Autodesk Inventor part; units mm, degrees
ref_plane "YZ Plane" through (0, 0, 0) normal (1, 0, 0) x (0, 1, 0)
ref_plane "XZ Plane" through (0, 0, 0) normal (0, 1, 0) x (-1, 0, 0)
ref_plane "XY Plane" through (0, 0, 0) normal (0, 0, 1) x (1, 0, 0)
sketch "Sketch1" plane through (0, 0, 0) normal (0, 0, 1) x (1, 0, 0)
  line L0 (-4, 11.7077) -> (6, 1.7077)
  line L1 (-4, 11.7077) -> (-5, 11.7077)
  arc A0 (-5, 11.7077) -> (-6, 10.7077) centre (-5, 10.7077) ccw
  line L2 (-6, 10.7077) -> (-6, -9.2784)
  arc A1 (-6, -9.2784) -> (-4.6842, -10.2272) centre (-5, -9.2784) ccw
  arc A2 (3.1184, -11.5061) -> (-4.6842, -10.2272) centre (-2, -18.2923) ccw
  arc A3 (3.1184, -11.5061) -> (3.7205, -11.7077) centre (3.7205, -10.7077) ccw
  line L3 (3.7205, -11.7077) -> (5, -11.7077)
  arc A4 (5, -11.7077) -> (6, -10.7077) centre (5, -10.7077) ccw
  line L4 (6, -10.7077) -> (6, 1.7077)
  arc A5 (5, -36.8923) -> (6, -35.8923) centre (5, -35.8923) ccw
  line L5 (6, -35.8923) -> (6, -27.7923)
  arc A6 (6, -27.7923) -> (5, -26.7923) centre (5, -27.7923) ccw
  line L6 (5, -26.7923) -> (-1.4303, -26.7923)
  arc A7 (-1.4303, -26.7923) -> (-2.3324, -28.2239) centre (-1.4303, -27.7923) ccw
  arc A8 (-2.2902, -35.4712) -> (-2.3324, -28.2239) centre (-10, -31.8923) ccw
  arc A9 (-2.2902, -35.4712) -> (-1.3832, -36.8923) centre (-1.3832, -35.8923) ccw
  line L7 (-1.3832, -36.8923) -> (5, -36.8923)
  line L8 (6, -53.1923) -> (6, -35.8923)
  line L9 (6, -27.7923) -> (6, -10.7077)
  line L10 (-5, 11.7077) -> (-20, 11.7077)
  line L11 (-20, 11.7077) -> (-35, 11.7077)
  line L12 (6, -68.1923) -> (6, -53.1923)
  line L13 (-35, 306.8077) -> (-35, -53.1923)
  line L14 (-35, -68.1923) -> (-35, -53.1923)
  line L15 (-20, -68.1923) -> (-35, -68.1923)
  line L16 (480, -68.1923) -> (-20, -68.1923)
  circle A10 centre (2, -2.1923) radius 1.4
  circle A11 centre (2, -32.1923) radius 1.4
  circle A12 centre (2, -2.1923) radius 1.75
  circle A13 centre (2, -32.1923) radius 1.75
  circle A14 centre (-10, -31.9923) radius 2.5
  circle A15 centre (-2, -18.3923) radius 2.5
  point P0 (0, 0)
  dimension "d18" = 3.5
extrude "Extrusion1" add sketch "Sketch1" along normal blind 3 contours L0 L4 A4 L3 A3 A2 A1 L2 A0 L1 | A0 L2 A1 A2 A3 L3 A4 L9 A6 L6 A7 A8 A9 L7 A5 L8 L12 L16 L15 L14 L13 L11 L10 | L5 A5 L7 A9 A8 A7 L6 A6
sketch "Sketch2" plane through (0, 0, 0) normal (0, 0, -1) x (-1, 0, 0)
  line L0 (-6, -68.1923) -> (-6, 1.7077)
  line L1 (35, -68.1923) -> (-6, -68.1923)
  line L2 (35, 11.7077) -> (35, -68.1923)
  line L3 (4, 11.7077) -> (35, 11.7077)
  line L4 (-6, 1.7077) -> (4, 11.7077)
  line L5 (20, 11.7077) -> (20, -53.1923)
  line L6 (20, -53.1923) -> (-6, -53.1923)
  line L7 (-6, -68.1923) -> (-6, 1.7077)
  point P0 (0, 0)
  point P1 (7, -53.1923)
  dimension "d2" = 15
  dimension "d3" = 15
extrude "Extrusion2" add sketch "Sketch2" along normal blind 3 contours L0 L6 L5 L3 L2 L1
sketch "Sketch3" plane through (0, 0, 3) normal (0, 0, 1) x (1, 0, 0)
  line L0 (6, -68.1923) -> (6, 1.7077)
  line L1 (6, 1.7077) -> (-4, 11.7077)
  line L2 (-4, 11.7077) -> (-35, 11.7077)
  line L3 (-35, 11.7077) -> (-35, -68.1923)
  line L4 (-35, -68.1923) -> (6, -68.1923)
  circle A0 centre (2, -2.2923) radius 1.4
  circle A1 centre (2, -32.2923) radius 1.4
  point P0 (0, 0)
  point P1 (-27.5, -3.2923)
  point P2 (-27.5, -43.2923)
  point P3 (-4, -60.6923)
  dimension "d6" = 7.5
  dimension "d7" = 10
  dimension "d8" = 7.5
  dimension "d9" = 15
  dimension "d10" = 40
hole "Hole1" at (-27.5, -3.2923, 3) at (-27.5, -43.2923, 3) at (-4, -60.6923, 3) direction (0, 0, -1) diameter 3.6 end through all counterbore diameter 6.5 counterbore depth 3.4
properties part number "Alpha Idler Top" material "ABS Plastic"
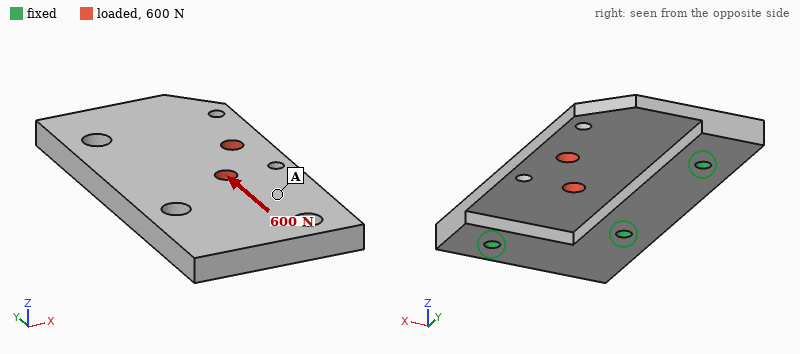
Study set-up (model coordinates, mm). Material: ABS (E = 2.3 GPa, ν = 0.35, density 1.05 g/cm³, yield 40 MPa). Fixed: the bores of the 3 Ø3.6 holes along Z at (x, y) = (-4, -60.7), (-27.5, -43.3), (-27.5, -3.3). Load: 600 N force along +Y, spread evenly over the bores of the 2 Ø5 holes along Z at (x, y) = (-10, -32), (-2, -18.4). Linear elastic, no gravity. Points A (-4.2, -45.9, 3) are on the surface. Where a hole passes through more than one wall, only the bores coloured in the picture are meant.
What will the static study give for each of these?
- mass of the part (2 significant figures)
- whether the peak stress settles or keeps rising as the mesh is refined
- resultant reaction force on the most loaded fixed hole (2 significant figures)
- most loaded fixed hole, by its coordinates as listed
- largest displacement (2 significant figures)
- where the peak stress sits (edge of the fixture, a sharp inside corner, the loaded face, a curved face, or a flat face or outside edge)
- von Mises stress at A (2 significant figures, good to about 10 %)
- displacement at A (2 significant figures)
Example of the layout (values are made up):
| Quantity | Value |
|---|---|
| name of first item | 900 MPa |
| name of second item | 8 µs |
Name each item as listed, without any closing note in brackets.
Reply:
| Quantity | Value |
|---|---|
| mass of the part | 15 g |
| whether the peak stress settles or keeps rising as the mesh is refined | keeps rising |
| resultant reaction force on the most loaded fixed hole | 260 N |
| most loaded fixed hole, by its coordinates as listed | (-27.5, -3.3) |
| largest displacement | 0.18 mm |
| where the peak stress sits | edge of the fixture |
| von Mises stress at A | 2.6 MPa |
| displacement at A | 0.12 mm |
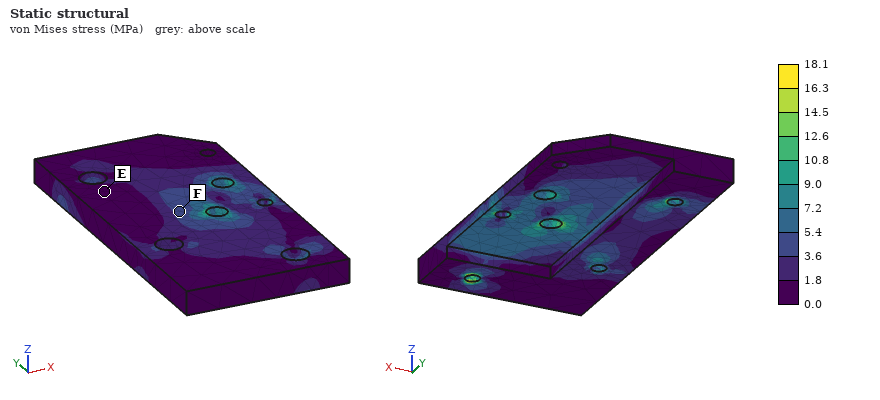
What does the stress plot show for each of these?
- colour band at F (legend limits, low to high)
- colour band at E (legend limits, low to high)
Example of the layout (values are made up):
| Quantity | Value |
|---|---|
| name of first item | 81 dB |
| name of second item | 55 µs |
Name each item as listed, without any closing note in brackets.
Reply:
| Quantity | Value |
|---|---|
| colour band at F | 3.6 to 5.4 MPa |
| colour band at E | 0.0 to 1.8 MPa |
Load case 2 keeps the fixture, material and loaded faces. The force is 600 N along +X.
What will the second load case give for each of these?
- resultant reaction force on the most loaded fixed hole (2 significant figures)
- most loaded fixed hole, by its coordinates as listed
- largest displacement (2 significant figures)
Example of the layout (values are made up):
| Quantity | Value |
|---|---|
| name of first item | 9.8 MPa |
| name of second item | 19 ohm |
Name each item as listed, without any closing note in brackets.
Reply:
| Quantity | Value |
|---|---|
| resultant reaction force on the most loaded fixed hole | 280 N |
| most loaded fixed hole, by its coordinates as listed | (-27.5, -43.3) |
| largest displacement | 0.49 mm |
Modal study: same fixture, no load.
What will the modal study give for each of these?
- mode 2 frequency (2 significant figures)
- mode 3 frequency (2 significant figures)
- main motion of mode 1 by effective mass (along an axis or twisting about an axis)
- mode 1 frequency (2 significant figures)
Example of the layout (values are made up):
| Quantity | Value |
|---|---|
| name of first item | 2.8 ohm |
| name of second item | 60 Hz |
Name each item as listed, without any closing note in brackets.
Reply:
| Quantity | Value |
|---|---|
| mode 2 frequency | 1700 Hz |
| mode 3 frequency | 2400 Hz |
| main motion of mode 1 by effective mass | along Z |
| mode 1 frequency | 920 Hz |
